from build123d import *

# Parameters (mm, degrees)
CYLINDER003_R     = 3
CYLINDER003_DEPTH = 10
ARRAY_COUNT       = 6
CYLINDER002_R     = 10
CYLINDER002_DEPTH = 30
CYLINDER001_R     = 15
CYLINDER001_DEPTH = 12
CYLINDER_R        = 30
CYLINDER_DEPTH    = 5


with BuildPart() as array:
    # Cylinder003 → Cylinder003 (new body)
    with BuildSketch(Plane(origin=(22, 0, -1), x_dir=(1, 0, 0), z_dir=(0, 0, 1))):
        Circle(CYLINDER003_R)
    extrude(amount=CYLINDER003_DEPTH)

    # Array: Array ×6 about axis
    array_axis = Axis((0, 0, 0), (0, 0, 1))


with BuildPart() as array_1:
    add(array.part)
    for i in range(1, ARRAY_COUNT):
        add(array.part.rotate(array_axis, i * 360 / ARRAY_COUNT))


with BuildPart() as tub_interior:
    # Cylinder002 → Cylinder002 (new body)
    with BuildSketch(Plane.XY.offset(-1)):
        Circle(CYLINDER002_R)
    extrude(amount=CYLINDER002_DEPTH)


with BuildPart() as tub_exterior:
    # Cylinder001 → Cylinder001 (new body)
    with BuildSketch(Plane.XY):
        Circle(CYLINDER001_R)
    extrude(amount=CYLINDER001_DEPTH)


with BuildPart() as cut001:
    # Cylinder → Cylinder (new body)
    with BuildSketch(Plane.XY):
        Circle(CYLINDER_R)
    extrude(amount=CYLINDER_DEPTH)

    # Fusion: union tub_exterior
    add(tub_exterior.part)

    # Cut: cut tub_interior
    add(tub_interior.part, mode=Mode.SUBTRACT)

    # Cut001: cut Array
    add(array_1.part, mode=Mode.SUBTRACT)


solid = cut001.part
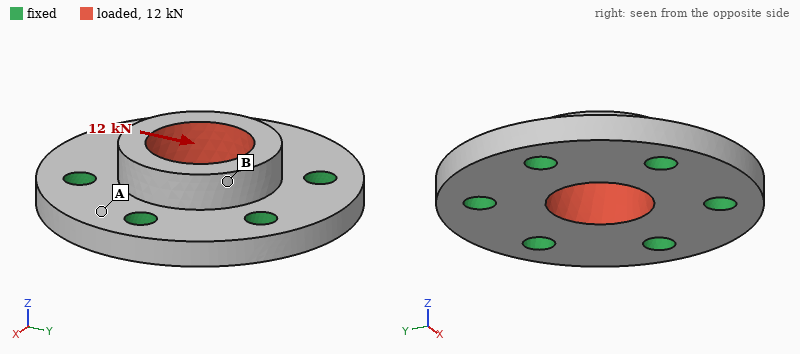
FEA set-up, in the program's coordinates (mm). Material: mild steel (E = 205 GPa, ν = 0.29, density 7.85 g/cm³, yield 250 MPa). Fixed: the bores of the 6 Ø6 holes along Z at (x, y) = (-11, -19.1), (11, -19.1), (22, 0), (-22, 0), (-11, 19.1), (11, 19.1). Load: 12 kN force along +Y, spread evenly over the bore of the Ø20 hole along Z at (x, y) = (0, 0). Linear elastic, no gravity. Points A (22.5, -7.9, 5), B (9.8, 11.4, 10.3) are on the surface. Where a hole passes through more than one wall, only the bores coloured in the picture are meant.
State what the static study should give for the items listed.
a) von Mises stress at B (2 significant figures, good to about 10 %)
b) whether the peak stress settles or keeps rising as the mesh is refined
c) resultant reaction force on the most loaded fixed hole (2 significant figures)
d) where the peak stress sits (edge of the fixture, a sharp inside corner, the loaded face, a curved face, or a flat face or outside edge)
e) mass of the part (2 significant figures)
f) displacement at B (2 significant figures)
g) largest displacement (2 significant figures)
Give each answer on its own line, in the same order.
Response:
18 MPa
keeps rising
2.5 kN
edge of the fixture
110 g
3.9 µm
5.7 µm
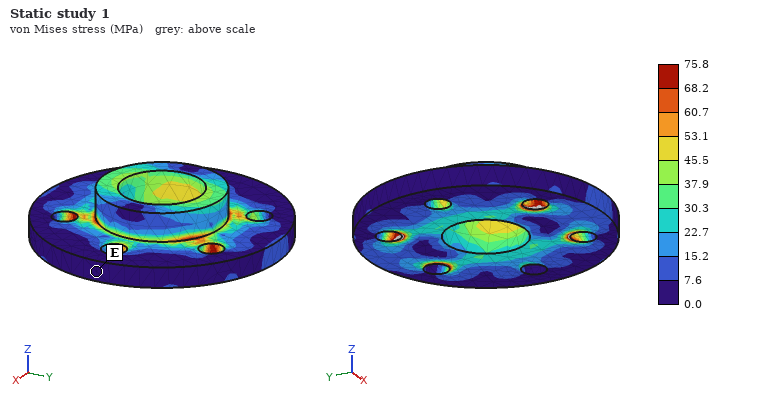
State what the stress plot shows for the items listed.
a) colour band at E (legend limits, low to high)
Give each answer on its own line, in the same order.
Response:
0.0 to 7.6 MPa
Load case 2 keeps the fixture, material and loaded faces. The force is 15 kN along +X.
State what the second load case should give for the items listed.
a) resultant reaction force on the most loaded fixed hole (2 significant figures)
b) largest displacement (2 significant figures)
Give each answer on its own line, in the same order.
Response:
3.5 kN
7.1 µm
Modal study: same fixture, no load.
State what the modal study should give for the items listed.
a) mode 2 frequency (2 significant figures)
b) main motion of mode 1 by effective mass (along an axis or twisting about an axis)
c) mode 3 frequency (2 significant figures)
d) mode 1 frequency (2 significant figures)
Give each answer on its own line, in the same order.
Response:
36 kHz
along Z
36 kHz
32 kHz
